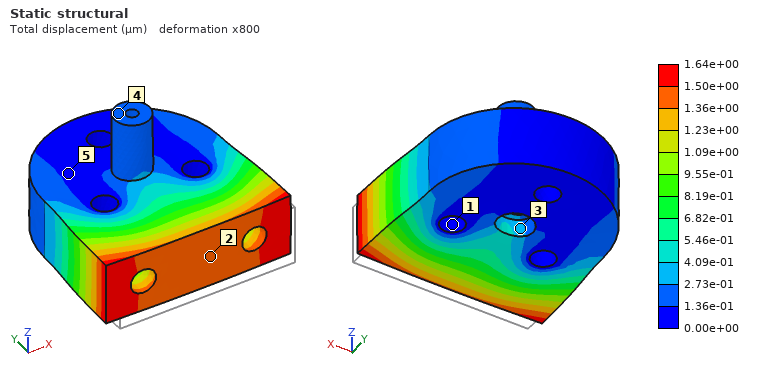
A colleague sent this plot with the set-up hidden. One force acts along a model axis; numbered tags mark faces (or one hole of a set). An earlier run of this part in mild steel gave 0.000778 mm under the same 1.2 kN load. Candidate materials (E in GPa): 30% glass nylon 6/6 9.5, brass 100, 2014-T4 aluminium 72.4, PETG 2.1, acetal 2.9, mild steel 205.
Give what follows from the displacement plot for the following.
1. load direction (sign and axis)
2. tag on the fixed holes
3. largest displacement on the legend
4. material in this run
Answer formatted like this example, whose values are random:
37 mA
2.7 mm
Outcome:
+Y
1
1.64e+00 µm
brass
